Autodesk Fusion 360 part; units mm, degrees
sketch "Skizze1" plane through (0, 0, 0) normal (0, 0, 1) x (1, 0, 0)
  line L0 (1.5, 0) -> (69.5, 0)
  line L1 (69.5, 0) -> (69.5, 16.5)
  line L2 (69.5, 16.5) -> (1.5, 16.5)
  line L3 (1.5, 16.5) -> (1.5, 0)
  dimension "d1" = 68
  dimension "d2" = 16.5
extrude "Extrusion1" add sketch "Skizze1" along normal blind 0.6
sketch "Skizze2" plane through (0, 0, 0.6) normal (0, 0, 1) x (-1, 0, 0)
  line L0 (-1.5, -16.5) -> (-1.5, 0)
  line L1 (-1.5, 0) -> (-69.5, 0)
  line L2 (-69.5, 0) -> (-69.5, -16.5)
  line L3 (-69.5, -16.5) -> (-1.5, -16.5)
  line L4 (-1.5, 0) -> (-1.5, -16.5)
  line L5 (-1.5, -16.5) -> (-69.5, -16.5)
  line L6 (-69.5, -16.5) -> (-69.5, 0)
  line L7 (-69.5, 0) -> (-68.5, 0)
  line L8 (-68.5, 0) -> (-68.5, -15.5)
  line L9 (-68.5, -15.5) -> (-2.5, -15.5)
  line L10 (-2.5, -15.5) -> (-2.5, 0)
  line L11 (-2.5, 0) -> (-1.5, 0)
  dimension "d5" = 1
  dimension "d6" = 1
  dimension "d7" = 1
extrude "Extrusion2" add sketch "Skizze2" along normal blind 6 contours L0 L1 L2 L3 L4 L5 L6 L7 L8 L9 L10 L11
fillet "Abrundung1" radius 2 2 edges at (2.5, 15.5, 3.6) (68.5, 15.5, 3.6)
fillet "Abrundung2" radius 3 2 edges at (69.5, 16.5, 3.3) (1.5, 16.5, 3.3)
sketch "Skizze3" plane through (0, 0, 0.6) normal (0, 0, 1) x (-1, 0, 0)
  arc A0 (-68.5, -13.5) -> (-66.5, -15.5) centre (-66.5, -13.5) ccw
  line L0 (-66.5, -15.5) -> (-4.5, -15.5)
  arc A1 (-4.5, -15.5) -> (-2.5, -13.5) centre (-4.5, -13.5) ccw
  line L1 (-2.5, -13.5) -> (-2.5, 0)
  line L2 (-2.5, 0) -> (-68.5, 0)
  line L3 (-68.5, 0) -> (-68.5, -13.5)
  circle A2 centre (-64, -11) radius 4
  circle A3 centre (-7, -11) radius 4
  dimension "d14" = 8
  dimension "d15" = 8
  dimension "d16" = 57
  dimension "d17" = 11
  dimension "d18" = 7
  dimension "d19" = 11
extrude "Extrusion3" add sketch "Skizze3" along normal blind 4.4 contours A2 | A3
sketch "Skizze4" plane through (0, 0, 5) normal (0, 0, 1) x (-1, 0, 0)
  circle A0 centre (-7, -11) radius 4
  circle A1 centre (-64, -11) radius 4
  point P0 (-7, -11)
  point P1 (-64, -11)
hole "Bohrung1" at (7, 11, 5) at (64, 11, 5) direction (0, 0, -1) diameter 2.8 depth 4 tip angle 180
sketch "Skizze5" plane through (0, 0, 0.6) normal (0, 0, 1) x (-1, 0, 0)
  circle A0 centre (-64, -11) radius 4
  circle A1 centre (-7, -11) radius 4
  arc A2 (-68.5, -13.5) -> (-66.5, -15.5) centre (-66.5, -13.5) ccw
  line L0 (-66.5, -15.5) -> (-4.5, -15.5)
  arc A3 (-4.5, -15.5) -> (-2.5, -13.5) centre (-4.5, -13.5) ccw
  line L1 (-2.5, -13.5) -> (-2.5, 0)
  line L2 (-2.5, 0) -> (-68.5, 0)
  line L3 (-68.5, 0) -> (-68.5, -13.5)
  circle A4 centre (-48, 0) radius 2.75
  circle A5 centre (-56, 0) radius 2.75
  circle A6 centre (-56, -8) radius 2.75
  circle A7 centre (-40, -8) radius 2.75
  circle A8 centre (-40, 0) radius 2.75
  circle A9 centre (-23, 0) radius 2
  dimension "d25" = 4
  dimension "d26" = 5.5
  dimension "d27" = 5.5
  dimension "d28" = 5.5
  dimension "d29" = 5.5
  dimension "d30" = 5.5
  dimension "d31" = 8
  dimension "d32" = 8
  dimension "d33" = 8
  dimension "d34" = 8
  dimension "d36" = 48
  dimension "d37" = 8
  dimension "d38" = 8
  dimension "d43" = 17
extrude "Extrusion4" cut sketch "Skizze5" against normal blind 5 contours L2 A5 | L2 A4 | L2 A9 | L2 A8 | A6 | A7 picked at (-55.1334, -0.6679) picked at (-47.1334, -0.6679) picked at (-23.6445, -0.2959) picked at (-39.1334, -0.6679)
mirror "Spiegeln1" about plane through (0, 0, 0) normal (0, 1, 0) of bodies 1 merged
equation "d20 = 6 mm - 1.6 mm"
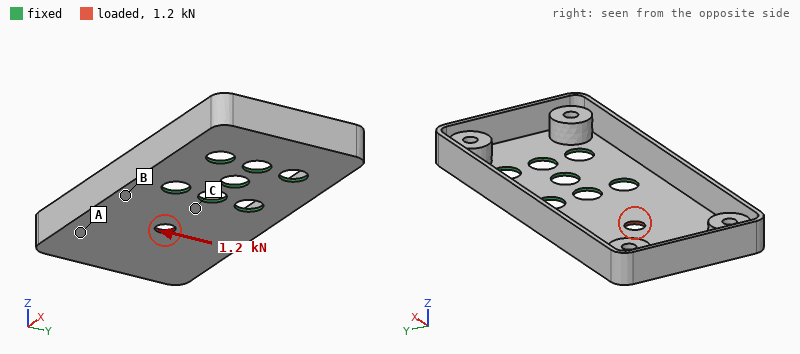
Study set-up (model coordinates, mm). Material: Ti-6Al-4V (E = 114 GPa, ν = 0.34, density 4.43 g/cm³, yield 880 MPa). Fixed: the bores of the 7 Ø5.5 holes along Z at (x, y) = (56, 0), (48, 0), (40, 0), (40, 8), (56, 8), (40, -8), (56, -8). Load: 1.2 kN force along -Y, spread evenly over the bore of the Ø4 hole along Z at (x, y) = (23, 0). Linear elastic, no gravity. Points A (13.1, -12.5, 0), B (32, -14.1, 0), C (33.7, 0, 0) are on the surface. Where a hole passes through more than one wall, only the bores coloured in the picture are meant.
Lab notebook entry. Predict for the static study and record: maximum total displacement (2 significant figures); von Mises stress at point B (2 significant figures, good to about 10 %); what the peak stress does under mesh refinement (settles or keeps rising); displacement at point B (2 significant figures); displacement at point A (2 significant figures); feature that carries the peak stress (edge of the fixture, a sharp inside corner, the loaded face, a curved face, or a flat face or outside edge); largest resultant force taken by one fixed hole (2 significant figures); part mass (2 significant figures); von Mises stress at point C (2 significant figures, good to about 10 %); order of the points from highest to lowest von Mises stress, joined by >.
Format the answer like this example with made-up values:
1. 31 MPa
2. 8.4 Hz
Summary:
1. 0.11 mm
2. 74 MPa
3. keeps rising
4. 0.020 mm
5. 0.059 mm
6. edge of the fixture
7. 800 N
8. 14 g
9. 140 MPa
10. C > B > A
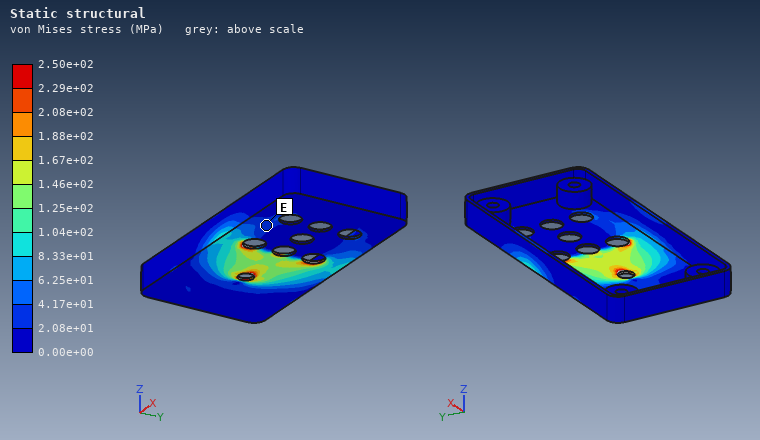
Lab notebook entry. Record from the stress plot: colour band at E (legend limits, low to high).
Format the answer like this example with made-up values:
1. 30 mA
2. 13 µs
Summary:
1. 2.08e+01 to 4.17e+01 MPa
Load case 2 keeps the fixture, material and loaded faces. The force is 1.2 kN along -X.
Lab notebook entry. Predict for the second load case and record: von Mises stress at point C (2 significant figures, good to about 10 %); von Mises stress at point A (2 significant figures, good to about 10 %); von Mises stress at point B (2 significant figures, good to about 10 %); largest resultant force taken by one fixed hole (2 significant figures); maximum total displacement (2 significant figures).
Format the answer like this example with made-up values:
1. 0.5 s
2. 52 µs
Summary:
1. 96 MPa
2. 21 MPa
3. 25 MPa
4. 400 N
5. 35 µm
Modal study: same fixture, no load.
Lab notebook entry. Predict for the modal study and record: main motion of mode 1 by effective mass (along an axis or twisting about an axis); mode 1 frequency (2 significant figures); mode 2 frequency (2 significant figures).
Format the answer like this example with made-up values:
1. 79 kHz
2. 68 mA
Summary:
1. along Z
2. 940 Hz
3. 1200 Hz
